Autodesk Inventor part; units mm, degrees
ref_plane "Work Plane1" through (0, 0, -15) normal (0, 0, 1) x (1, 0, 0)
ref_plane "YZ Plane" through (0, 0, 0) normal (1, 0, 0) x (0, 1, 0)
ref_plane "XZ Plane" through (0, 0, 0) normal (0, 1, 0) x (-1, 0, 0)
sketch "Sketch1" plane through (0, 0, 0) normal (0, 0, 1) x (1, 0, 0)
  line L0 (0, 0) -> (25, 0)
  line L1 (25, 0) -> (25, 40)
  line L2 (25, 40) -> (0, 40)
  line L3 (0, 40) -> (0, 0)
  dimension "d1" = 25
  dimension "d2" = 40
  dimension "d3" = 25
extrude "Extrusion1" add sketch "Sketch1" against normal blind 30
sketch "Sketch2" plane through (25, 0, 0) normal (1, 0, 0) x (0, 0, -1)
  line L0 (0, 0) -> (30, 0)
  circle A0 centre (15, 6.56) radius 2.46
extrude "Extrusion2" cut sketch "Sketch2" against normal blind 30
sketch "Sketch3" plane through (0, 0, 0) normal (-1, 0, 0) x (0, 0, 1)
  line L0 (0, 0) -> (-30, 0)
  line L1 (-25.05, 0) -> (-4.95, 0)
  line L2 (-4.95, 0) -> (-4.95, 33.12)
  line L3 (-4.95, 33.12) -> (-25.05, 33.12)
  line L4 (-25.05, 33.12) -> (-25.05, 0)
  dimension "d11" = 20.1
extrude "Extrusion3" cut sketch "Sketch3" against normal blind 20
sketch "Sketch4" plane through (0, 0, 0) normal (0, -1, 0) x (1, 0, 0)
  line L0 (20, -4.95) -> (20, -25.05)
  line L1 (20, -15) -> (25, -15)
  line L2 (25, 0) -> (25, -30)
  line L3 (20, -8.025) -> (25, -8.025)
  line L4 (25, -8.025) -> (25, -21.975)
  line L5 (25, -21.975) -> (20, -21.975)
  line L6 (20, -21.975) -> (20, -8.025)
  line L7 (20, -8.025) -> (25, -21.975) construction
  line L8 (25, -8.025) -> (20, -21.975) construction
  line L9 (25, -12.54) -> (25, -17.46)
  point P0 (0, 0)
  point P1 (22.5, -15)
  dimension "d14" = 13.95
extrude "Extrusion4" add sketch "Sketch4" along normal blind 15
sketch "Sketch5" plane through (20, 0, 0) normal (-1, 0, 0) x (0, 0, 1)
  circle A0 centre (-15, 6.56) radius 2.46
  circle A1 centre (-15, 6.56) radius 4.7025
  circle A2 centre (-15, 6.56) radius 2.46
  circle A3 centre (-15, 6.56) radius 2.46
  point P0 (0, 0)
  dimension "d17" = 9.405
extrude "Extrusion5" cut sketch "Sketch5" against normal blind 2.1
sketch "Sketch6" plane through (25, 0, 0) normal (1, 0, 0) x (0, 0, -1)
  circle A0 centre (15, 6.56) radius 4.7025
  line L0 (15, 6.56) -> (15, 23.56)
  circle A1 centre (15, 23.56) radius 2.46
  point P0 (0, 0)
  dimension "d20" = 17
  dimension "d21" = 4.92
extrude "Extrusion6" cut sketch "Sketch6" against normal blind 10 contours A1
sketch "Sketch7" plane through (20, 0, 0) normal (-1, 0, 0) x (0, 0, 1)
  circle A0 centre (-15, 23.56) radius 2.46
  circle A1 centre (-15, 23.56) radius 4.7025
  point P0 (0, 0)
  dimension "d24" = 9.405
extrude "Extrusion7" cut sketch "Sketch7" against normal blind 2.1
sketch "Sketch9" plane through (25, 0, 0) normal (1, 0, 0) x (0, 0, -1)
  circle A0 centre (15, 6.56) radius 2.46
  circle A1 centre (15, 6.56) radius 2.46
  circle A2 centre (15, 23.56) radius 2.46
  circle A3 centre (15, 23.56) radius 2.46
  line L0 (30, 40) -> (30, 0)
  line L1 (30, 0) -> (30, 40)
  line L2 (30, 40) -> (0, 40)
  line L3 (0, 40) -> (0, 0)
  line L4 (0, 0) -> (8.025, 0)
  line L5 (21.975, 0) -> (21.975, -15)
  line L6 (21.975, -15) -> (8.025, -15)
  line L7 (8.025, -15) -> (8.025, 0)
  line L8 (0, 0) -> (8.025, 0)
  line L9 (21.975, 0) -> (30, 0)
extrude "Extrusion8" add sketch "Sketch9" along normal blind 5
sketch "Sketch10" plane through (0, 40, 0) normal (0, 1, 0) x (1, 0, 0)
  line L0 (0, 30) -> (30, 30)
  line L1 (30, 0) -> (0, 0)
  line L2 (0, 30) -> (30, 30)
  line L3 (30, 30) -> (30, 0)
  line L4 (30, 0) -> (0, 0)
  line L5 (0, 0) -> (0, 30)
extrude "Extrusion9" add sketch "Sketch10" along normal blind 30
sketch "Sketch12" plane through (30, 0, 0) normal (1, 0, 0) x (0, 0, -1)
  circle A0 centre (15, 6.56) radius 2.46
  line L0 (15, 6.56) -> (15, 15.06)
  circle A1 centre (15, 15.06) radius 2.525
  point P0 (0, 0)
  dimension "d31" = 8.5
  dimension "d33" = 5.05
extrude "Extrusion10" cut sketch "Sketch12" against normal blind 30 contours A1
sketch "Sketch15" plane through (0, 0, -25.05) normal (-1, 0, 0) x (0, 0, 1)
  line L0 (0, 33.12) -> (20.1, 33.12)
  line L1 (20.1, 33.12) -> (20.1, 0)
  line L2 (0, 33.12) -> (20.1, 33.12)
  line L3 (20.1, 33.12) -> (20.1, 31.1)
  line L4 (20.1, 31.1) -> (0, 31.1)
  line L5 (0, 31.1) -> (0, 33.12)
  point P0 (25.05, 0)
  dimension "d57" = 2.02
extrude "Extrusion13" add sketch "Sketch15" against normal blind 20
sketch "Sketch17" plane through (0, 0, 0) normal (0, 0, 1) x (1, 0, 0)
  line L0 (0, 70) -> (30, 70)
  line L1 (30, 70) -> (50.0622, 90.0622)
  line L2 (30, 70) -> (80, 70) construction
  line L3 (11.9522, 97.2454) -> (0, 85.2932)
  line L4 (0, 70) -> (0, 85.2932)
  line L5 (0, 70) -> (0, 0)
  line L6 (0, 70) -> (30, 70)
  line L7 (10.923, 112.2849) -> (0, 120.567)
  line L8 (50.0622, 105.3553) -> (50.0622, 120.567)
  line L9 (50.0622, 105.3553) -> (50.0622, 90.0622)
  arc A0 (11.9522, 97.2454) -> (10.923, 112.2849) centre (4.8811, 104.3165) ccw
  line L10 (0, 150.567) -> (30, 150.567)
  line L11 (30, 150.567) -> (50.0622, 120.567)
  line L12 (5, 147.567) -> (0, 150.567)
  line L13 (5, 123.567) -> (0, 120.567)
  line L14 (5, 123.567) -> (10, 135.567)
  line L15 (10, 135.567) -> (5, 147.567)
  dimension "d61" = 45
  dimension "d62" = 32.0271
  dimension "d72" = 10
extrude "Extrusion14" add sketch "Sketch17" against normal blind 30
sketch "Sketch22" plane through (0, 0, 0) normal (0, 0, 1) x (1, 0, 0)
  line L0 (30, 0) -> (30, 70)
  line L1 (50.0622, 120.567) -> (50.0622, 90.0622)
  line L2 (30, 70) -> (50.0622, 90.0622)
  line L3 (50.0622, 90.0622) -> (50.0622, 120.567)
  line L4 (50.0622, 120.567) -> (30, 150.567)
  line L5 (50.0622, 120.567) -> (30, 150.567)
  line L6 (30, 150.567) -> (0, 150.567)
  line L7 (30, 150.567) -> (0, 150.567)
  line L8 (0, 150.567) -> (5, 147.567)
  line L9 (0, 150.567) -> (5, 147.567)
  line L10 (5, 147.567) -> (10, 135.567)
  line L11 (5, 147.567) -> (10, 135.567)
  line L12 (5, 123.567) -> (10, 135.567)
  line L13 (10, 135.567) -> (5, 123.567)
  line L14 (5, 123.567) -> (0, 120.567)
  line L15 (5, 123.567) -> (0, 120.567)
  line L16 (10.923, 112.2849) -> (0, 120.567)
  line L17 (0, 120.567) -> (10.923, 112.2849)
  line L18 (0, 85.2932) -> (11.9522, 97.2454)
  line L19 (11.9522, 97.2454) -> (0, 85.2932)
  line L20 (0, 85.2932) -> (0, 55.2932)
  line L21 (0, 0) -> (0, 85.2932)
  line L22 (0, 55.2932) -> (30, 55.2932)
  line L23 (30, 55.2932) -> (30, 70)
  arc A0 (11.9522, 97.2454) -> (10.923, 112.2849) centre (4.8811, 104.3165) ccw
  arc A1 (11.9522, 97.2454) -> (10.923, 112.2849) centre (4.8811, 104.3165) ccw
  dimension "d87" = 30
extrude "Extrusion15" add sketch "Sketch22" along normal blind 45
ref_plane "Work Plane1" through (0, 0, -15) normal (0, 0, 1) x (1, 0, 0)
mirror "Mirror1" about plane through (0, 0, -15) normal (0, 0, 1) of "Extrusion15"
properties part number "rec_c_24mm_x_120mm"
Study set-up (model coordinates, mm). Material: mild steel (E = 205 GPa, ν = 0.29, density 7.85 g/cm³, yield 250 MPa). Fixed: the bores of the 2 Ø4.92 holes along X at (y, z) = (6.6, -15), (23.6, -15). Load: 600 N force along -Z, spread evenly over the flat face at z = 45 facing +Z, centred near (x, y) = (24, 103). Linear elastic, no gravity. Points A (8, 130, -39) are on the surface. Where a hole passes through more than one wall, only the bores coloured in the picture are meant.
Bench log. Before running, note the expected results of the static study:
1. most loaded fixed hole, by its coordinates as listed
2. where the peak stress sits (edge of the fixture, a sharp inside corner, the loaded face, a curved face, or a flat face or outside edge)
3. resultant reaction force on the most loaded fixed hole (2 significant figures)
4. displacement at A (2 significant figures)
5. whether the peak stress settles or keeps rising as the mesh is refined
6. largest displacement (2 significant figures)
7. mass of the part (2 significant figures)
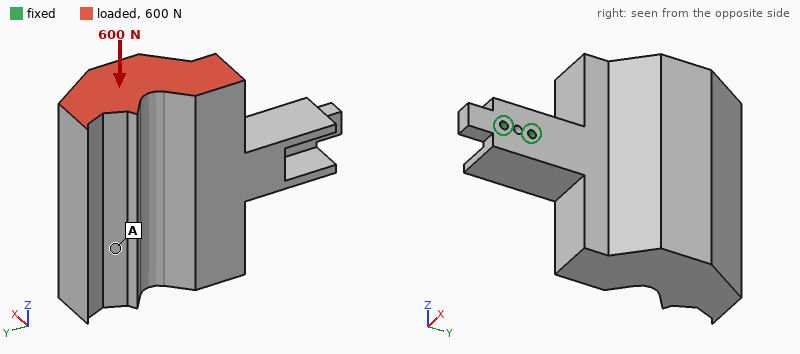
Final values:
(23.6, -15)
edge of the fixture
2.6 kN
33 µm
keeps rising
46 µm
3.6 kg
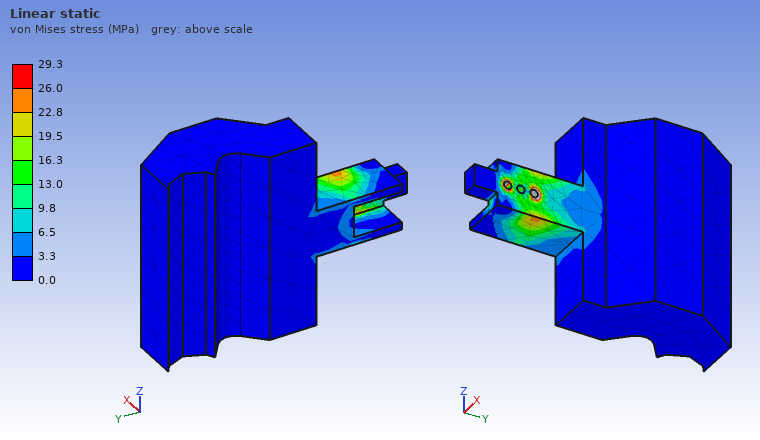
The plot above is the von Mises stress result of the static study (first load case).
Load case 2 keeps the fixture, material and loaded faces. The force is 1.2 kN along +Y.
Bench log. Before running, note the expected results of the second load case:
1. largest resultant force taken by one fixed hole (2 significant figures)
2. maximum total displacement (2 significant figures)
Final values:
3.2 kN
77 µm
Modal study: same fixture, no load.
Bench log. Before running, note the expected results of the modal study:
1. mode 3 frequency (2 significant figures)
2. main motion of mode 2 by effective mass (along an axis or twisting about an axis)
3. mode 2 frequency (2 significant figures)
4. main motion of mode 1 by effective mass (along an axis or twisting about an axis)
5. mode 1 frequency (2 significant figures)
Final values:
560 Hz
along Z
370 Hz
along X
350 Hz
